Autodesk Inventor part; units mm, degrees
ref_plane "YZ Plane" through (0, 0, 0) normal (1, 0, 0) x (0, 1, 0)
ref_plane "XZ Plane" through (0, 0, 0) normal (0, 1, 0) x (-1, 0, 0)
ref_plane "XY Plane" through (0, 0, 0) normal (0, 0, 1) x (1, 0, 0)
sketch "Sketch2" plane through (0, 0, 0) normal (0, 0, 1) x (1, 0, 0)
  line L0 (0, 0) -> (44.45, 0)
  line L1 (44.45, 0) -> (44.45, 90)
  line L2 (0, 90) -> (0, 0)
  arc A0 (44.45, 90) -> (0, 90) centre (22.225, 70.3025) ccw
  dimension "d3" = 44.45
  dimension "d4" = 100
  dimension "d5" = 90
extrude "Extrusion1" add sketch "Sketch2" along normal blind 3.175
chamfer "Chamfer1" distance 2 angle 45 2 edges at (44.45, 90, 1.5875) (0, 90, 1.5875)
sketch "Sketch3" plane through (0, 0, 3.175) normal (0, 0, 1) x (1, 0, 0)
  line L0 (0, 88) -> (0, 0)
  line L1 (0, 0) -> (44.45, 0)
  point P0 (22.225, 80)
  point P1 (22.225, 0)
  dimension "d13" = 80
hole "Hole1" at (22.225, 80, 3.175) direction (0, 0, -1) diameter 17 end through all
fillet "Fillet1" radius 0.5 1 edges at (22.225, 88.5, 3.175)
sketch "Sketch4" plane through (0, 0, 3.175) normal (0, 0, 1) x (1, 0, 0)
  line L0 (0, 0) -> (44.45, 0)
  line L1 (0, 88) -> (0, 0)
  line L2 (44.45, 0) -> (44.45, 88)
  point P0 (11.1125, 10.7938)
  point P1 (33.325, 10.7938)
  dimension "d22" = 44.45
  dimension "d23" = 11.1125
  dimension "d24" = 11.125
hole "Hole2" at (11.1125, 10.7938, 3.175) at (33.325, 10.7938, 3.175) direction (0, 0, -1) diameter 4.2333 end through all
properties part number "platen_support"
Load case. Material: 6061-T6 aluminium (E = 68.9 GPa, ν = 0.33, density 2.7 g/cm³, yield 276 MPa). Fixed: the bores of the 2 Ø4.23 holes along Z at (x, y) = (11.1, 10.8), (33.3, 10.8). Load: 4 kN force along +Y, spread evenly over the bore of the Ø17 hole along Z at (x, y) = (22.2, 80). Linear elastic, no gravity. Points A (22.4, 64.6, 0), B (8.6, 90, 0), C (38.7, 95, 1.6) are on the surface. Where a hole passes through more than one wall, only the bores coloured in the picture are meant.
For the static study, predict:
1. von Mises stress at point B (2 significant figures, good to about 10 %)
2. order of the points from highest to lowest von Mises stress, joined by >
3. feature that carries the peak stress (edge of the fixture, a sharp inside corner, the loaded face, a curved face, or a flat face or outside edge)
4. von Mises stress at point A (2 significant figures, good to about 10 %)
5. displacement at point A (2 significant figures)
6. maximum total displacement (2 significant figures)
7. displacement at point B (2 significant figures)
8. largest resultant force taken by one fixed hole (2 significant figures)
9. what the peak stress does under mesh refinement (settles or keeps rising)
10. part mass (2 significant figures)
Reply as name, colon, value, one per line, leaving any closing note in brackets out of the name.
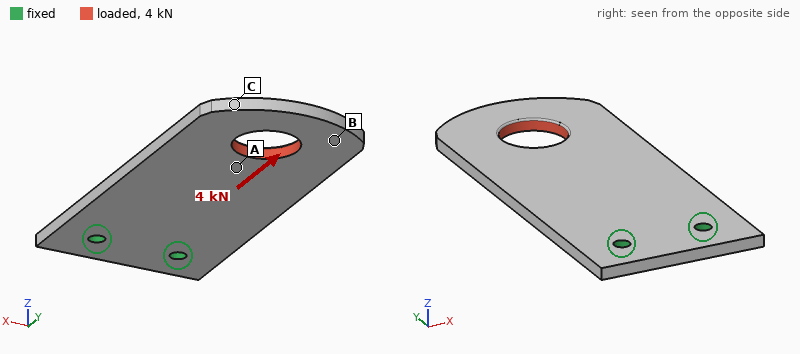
von Mises stress at point B: 21 MPa
order of the points from highest to lowest von Mises stress, joined by >: A > B > C
feature that carries the peak stress: edge of the fixture
von Mises stress at point A: 40 MPa
displacement at point A: 0.18 mm
maximum total displacement: 0.47 mm
displacement at point B: 0.37 mm
largest resultant force taken by one fixed hole: 2.0 kN
what the peak stress does under mesh refinement: keeps rising
part mass: 35 g
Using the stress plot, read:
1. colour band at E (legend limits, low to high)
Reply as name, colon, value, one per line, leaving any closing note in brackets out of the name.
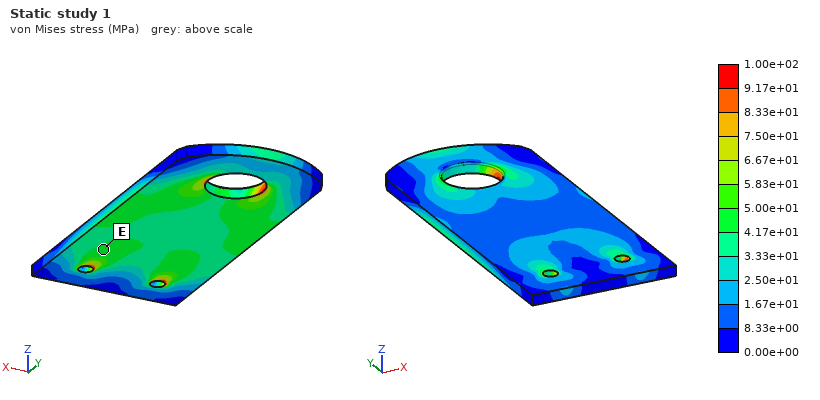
colour band at E: 4.17e+01 to 5.00e+01 MPa
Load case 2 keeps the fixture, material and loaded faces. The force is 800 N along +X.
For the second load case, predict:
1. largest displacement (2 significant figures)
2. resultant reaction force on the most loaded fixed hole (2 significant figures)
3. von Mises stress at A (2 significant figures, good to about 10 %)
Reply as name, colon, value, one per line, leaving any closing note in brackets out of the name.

largest displacement: 0.13 mm
resultant reaction force on the most loaded fixed hole: 2.3 kN
von Mises stress at A: 23 MPa
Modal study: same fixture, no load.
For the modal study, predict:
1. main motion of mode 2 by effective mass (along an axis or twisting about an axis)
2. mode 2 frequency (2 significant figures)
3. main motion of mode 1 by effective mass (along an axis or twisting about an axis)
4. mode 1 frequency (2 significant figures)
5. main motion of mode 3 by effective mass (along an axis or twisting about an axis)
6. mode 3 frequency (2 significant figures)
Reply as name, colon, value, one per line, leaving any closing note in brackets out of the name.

main motion of mode 2 by effective mass: twisting about Y
mode 2 frequency: 1500 Hz
main motion of mode 1 by effective mass: along Z
mode 1 frequency: 380 Hz
main motion of mode 3 by effective mass: along Z
mode 3 frequency: 2100 Hz
